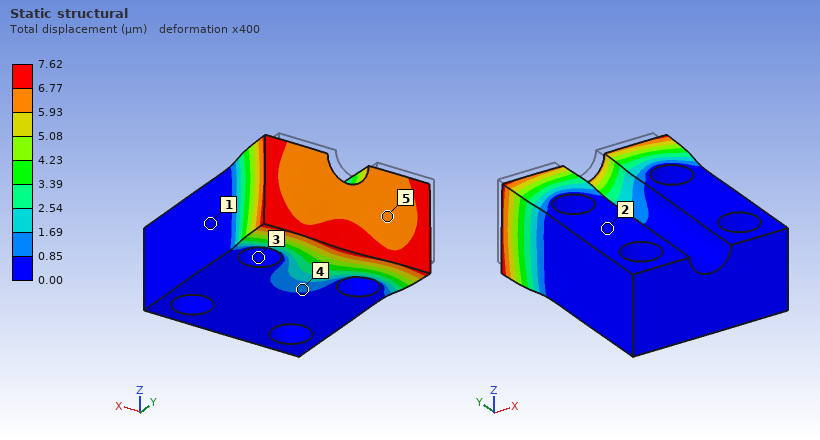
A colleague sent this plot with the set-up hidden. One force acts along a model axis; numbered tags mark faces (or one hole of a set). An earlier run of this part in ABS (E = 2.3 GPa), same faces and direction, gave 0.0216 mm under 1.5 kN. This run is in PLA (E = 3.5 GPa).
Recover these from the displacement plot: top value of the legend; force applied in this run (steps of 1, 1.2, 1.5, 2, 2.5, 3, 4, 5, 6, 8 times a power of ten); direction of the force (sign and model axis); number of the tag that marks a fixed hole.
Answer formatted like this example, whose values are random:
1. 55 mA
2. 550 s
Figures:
1. 7.62 µm
2. 800 N
3. -Y
4. 3
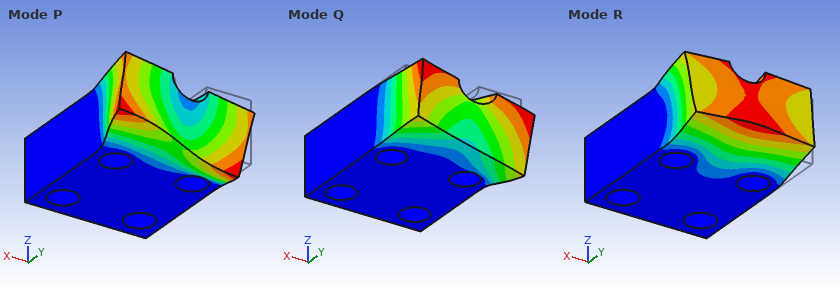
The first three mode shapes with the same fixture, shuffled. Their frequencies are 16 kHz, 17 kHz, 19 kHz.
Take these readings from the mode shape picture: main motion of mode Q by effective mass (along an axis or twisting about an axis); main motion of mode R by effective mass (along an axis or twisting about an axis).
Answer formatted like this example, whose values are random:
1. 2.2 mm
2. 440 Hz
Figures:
1. along X
2. along Z
